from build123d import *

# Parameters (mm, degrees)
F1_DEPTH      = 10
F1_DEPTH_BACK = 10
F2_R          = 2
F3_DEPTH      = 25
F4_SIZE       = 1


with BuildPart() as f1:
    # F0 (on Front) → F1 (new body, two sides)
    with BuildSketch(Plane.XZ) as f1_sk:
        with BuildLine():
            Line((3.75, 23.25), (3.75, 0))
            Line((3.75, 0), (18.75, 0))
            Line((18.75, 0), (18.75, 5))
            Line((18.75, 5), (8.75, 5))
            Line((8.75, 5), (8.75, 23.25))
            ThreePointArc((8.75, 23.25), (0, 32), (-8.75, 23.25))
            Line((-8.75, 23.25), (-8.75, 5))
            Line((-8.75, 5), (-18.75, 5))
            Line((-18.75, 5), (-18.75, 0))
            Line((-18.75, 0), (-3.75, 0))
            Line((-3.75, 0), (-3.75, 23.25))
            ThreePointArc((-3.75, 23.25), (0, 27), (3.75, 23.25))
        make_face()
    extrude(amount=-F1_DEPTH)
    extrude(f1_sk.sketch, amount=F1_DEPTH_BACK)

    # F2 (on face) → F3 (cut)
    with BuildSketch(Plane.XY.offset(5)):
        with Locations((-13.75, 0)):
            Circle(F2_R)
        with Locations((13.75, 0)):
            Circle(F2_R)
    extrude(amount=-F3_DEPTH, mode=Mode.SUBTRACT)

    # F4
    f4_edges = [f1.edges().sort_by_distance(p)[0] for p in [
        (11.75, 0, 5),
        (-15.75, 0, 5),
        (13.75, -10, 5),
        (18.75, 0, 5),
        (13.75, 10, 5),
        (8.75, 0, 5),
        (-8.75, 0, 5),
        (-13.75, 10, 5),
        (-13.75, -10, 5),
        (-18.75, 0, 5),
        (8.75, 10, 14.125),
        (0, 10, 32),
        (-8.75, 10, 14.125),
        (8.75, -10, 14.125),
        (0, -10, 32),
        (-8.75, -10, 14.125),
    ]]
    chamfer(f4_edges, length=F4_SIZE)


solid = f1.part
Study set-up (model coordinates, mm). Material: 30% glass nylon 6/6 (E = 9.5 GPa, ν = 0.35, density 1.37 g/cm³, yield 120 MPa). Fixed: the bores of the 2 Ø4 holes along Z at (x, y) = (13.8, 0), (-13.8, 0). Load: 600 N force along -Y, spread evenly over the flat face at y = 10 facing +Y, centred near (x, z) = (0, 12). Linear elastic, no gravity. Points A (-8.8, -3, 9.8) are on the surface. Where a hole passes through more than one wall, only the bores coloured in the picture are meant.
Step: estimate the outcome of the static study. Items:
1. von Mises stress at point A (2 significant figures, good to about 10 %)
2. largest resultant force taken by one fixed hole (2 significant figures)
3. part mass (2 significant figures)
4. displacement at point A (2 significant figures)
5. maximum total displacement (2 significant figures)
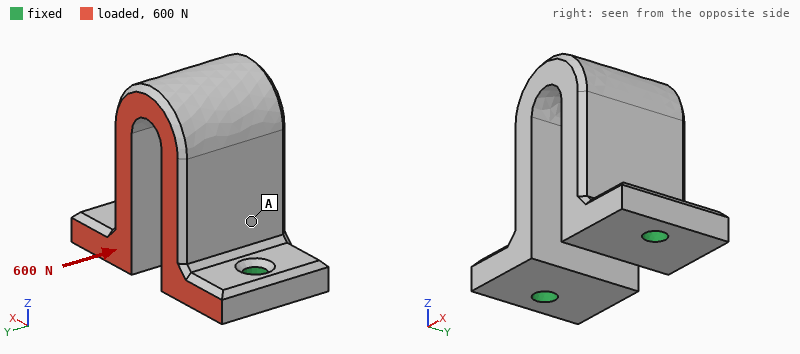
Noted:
8.1 MPa
300 N
11 g
0.085 mm
0.30 mm
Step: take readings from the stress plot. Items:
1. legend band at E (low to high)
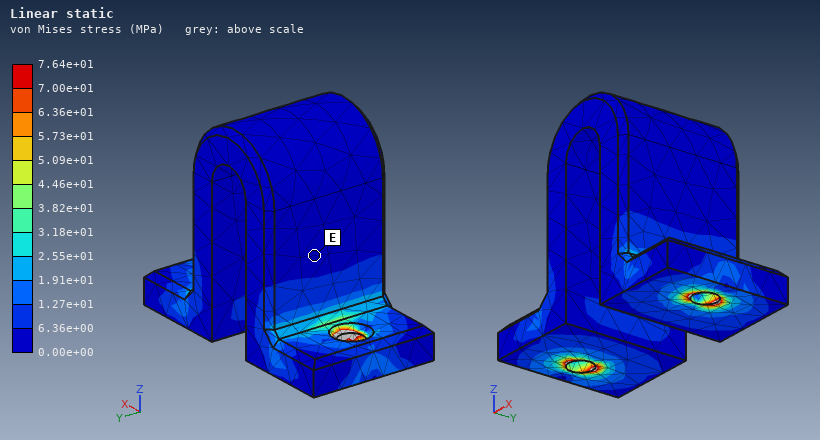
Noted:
0.00e+00 to 6.36e+00 MPa
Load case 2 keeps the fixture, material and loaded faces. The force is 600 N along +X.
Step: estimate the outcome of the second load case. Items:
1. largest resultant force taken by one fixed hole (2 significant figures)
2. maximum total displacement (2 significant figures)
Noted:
370 N
0.19 mm
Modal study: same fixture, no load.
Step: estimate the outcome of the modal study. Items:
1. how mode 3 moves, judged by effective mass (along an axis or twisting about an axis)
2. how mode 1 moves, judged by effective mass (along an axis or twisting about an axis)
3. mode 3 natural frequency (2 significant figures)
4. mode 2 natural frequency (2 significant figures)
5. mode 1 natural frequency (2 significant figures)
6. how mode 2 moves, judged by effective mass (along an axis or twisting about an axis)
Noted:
twisting about Z
along Y
6200 Hz
3800 Hz
2400 Hz
along X
